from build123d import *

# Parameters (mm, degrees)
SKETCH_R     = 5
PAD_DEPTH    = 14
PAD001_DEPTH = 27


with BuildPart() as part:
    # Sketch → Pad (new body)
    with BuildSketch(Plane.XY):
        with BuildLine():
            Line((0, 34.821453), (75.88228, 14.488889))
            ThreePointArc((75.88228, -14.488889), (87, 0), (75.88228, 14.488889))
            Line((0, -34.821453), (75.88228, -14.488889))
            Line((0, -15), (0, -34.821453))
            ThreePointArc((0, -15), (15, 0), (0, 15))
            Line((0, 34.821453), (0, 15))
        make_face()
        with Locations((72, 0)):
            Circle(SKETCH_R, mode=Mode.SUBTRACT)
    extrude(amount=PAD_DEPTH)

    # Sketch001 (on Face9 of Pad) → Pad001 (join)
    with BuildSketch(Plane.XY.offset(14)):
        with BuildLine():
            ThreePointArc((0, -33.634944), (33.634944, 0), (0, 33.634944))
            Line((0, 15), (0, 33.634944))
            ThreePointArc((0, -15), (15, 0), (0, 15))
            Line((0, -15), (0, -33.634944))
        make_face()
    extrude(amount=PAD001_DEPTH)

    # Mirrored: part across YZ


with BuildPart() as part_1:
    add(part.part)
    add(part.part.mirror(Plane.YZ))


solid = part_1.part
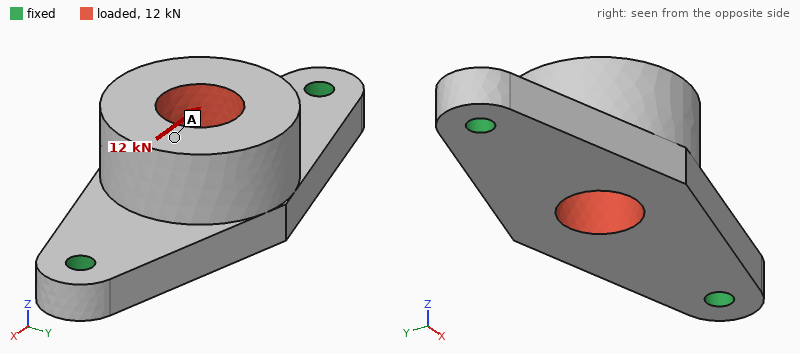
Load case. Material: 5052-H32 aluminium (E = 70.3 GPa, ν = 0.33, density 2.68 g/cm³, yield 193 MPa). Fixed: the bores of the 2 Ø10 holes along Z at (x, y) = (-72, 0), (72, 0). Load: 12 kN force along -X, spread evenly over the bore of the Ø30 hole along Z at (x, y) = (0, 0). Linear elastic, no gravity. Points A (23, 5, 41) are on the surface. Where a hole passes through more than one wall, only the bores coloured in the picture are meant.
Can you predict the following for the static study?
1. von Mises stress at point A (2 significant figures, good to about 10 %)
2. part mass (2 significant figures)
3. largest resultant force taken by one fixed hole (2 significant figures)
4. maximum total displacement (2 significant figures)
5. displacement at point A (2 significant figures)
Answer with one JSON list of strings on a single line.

["4.3 MPa", "470 g", "6.2 kN", "27 µm", "25 µm"]
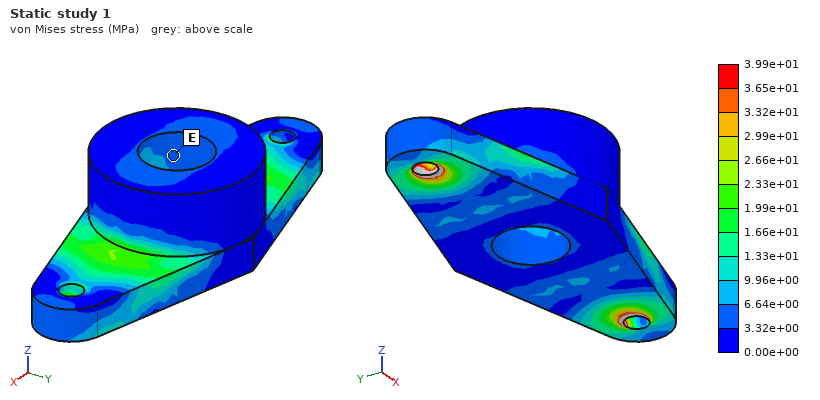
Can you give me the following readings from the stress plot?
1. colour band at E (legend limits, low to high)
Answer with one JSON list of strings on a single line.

["3.32e+00 to 6.64e+00 MPa"]
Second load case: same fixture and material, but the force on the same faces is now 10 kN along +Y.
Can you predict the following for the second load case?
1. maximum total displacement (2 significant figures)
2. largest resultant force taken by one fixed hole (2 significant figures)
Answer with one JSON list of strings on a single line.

["0.19 mm", "5.0 kN"]
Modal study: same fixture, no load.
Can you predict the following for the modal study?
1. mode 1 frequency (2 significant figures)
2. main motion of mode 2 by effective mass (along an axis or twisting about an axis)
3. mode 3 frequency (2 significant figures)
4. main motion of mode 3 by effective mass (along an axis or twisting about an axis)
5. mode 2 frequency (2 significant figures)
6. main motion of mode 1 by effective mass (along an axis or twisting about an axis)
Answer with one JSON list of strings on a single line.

["2100 Hz", "along Z", "5300 Hz", "along Y", "2800 Hz", "along Y"]
